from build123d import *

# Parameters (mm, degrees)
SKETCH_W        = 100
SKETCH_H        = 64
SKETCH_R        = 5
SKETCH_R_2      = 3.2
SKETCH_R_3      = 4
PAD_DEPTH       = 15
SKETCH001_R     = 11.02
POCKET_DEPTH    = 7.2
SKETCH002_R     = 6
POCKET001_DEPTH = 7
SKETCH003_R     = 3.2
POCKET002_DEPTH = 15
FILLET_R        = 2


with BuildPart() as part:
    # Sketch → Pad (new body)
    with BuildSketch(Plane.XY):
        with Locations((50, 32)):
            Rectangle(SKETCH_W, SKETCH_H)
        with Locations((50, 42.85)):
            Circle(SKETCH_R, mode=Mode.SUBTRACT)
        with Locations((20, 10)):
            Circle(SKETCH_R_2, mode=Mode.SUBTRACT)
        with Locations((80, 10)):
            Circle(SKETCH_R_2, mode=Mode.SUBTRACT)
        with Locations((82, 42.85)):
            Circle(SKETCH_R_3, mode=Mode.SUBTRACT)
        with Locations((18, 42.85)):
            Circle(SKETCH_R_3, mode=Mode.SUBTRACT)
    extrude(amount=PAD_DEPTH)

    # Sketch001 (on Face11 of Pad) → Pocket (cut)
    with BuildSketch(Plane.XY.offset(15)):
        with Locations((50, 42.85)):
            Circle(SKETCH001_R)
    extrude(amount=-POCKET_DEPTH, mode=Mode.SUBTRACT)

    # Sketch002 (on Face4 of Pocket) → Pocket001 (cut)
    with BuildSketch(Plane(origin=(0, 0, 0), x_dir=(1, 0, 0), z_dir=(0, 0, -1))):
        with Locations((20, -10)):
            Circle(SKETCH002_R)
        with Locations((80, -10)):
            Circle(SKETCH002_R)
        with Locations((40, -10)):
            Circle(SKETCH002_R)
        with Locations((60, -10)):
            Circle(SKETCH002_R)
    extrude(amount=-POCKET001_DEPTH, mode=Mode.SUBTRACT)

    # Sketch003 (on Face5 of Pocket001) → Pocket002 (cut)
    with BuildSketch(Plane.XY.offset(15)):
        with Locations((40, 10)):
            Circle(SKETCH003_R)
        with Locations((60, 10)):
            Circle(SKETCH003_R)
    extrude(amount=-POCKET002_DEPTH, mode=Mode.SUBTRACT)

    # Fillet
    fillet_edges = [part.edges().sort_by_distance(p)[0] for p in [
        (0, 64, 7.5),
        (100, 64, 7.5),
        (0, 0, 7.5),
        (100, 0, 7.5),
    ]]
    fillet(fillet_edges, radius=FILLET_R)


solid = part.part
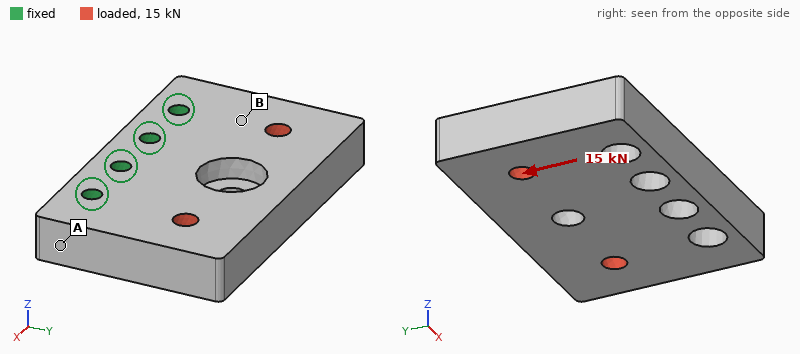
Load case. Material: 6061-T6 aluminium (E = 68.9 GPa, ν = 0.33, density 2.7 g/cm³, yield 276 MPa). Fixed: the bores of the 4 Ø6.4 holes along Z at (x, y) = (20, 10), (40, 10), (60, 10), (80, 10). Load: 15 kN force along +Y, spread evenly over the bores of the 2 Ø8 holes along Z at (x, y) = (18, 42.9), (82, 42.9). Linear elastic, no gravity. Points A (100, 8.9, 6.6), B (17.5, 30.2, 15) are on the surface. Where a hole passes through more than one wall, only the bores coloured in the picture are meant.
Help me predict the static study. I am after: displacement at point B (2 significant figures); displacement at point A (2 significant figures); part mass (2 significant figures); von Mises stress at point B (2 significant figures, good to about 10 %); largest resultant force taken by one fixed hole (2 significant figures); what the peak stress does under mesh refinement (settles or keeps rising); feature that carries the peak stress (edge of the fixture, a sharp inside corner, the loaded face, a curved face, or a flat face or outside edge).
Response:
13 µm
10 µm
230 g
21 MPa
4.9 kN
keeps rising
edge of the fixture
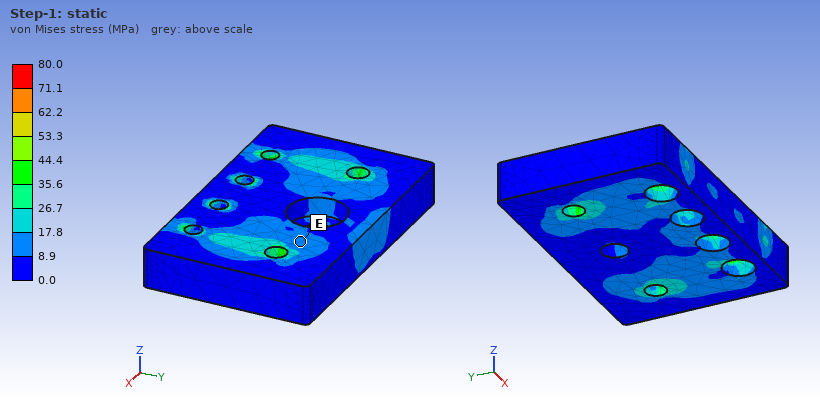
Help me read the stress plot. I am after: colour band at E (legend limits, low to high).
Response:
8.9 to 17.8 MPa
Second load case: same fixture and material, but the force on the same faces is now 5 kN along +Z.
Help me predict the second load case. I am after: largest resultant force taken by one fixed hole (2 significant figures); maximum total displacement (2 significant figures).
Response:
1.6 kN
0.16 mm
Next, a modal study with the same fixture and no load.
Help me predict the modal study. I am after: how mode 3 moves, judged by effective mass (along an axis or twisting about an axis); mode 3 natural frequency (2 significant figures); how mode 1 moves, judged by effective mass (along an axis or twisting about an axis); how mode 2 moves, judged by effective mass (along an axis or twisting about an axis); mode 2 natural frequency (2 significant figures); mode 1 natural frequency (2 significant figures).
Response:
along X
8200 Hz
along Z
twisting about Y
4300 Hz
2700 Hz
